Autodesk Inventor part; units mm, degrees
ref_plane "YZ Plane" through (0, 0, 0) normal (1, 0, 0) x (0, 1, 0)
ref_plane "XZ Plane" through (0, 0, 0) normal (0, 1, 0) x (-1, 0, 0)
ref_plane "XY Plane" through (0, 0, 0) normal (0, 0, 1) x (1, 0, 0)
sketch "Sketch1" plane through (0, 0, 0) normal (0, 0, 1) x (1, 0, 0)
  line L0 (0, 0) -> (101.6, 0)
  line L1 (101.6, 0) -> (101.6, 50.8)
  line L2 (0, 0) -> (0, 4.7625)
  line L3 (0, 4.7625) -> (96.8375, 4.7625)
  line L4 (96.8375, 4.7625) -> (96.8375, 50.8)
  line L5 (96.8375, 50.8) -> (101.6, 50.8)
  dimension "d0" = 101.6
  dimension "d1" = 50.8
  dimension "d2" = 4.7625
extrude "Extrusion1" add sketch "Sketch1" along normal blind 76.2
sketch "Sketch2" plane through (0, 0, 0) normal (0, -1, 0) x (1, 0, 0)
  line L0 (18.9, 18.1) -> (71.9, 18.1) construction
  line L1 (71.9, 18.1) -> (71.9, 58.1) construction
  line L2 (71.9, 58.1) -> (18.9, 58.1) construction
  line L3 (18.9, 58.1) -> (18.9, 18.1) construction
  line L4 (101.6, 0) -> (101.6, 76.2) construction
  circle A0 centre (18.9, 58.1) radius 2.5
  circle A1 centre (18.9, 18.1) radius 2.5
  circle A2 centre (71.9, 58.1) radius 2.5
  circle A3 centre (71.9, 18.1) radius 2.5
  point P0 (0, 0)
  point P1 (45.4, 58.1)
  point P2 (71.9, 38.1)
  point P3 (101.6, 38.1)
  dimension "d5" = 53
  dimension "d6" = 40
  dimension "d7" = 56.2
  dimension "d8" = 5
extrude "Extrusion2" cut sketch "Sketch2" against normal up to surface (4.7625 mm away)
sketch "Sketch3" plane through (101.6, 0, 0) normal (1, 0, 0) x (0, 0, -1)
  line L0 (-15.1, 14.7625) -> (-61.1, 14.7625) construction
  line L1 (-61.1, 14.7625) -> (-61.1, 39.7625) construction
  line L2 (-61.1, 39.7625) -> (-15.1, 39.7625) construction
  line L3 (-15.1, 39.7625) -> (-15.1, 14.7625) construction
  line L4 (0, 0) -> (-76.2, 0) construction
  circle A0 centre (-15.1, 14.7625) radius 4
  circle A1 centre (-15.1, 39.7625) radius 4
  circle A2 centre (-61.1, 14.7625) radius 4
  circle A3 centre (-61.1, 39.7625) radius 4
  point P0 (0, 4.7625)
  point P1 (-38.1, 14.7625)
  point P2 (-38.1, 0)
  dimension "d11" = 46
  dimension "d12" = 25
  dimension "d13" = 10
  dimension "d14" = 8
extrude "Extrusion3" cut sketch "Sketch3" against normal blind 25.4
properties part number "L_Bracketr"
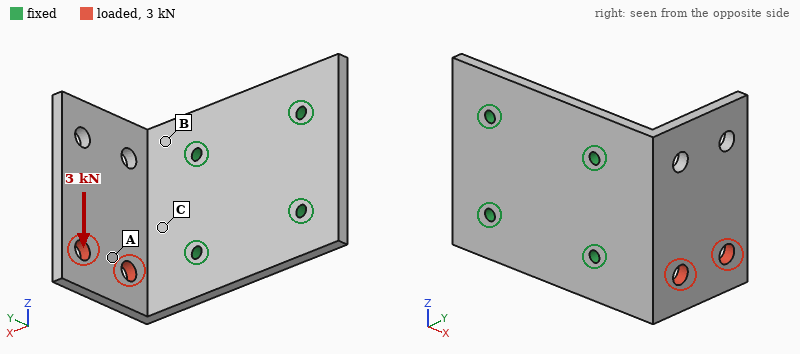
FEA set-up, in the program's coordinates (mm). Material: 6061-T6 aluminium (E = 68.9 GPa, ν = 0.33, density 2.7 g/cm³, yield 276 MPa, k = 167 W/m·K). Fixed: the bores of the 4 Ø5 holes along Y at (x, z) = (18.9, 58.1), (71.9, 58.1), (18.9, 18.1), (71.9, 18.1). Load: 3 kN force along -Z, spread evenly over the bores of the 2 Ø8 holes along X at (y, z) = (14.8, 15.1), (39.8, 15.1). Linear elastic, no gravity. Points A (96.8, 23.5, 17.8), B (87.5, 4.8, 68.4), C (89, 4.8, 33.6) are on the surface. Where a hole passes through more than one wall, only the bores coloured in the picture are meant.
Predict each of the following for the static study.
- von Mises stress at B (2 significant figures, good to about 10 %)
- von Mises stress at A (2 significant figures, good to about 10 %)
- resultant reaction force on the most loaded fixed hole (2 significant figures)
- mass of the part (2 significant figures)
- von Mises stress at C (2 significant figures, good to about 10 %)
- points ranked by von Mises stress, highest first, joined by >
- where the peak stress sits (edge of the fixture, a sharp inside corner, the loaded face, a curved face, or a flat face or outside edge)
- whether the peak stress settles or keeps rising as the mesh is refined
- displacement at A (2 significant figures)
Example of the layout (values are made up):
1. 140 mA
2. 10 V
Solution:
1. 70 MPa
2. 30 MPa
3. 2.7 kN
4. 140 g
5. 120 MPa
6. C > B > A
7. edge of the fixture
8. keeps rising
9. 0.33 mm
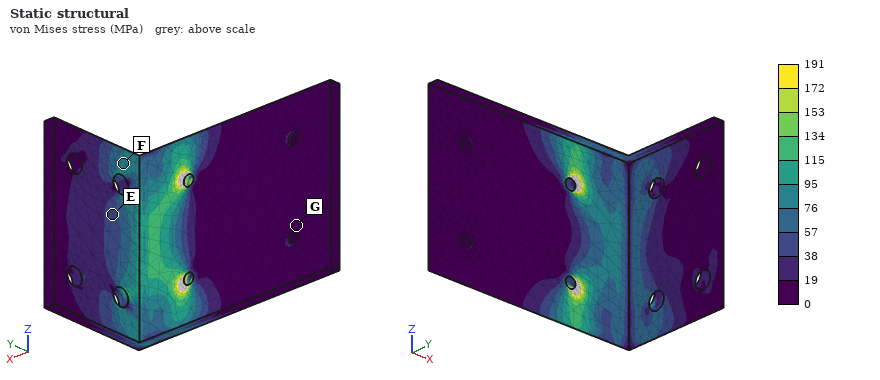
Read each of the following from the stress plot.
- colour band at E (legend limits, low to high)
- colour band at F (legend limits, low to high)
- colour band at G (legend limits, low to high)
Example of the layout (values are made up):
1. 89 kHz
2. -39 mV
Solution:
1. 38 to 57 MPa
2. 76 to 95 MPa
3. 0 to 19 MPa
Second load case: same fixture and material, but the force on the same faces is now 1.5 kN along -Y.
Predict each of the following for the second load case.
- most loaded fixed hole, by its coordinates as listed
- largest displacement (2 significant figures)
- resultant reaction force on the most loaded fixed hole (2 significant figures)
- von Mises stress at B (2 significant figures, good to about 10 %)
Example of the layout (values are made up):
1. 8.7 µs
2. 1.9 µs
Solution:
1. (71.9, 18.1)
2. 0.88 mm
3. 1.6 kN
4. 57 MPa
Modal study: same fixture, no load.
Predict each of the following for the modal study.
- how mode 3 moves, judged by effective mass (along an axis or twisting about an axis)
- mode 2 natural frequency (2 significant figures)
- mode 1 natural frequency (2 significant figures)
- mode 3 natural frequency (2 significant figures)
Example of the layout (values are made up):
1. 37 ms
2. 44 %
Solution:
1. along Y
2. 1600 Hz
3. 880 Hz
4. 2700 Hz
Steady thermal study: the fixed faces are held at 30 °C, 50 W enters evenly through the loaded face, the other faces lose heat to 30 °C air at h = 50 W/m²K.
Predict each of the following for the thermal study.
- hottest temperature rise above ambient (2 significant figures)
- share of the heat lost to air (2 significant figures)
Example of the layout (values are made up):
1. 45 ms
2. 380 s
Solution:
1. 52 K
2. 30 %
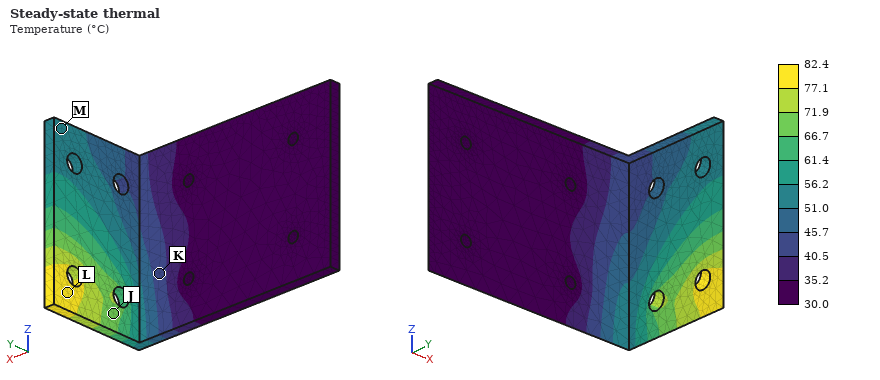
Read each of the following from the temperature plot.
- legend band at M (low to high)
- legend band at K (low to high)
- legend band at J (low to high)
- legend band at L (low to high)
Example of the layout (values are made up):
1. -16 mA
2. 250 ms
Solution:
1. 51.0 to 56.2 °C
2. 40.5 to 45.7 °C
3. 66.7 to 71.9 °C
4. 77.1 to 82.4 °C
